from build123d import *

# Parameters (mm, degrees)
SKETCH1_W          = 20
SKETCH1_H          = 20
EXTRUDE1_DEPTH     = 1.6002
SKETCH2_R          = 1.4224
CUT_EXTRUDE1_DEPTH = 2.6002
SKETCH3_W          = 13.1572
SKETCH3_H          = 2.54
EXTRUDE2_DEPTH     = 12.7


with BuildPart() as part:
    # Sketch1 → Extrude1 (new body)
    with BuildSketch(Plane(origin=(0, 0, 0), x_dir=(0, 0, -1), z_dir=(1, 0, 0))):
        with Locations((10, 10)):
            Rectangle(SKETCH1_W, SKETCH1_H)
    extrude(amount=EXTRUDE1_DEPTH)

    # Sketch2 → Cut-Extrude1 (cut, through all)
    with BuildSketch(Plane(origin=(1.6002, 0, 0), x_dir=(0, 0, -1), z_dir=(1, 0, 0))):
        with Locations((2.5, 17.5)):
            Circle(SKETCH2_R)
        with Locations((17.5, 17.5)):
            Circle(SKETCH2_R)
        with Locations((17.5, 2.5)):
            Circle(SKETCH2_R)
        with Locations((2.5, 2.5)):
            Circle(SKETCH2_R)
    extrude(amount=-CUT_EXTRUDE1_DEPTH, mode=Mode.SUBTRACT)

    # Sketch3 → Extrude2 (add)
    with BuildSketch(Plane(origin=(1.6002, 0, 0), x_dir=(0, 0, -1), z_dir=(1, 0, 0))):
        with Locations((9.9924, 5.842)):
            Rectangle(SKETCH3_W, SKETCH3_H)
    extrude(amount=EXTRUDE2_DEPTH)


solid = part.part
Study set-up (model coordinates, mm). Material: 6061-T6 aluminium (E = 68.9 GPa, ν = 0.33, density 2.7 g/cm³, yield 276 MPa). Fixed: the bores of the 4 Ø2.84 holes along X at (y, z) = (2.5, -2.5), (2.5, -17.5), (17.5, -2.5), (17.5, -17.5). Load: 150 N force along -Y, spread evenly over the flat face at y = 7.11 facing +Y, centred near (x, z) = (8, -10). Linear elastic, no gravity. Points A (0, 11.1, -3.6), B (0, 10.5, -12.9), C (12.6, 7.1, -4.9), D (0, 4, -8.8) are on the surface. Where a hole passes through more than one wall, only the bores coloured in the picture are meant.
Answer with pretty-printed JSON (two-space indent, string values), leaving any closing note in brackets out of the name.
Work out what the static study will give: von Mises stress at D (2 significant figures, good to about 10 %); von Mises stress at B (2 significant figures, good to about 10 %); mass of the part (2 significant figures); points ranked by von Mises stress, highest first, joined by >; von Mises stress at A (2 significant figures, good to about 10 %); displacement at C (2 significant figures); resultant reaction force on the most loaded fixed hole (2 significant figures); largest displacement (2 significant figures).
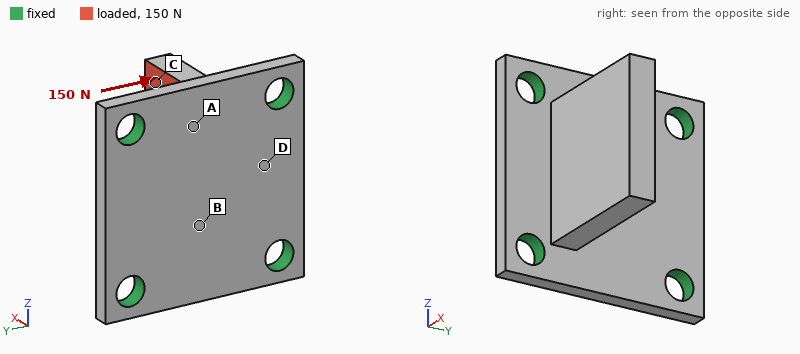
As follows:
{
  "von Mises stress at D": "36 MPa",
  "von Mises stress at B": "24 MPa",
  "mass of the part": "2.8 g",
  "points ranked by von Mises stress, highest first, joined by >": "D > B > A > C",
  "von Mises stress at A": "15 MPa",
  "displacement at C": "59 µm",
  "resultant reaction force on the most loaded fixed hole": "66 N",
  "largest displacement": "70 µm"
}
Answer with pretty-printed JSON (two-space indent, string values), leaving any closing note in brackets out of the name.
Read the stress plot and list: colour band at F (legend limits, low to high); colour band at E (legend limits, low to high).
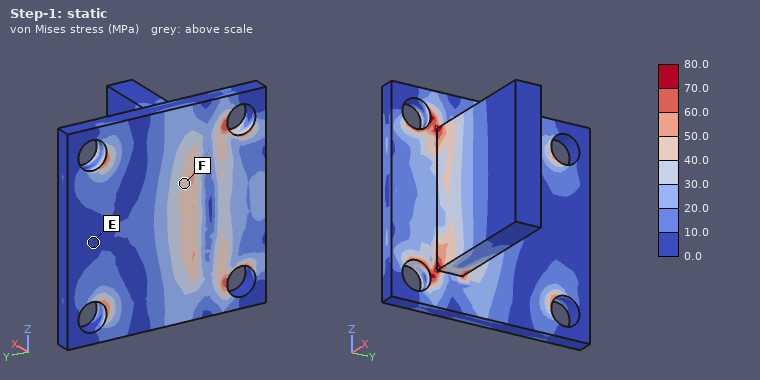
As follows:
{
  "colour band at F": "40.0 to 50.0 MPa",
  "colour band at E": "0.0 to 10.0 MPa"
}
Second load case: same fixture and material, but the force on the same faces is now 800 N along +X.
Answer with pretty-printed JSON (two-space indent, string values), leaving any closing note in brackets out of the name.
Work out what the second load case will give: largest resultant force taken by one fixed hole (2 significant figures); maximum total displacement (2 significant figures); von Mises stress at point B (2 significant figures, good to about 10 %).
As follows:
{
  "largest resultant force taken by one fixed hole": "320 N",
  "maximum total displacement": "0.12 mm",
  "von Mises stress at point B": "55 MPa"
}
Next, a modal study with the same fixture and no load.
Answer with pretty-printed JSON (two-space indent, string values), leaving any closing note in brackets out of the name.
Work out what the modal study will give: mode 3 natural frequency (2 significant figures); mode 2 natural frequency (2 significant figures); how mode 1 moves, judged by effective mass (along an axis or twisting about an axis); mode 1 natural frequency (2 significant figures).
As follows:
{
  "mode 3 natural frequency": "26 kHz",
  "mode 2 natural frequency": "23 kHz",
  "how mode 1 moves, judged by effective mass": "along Y",
  "mode 1 natural frequency": "8400 Hz"
}
